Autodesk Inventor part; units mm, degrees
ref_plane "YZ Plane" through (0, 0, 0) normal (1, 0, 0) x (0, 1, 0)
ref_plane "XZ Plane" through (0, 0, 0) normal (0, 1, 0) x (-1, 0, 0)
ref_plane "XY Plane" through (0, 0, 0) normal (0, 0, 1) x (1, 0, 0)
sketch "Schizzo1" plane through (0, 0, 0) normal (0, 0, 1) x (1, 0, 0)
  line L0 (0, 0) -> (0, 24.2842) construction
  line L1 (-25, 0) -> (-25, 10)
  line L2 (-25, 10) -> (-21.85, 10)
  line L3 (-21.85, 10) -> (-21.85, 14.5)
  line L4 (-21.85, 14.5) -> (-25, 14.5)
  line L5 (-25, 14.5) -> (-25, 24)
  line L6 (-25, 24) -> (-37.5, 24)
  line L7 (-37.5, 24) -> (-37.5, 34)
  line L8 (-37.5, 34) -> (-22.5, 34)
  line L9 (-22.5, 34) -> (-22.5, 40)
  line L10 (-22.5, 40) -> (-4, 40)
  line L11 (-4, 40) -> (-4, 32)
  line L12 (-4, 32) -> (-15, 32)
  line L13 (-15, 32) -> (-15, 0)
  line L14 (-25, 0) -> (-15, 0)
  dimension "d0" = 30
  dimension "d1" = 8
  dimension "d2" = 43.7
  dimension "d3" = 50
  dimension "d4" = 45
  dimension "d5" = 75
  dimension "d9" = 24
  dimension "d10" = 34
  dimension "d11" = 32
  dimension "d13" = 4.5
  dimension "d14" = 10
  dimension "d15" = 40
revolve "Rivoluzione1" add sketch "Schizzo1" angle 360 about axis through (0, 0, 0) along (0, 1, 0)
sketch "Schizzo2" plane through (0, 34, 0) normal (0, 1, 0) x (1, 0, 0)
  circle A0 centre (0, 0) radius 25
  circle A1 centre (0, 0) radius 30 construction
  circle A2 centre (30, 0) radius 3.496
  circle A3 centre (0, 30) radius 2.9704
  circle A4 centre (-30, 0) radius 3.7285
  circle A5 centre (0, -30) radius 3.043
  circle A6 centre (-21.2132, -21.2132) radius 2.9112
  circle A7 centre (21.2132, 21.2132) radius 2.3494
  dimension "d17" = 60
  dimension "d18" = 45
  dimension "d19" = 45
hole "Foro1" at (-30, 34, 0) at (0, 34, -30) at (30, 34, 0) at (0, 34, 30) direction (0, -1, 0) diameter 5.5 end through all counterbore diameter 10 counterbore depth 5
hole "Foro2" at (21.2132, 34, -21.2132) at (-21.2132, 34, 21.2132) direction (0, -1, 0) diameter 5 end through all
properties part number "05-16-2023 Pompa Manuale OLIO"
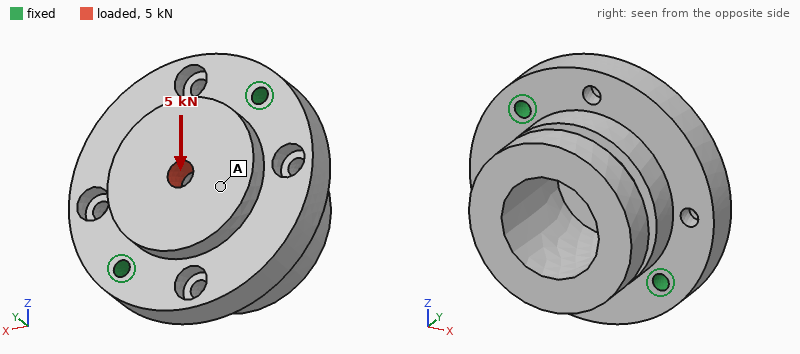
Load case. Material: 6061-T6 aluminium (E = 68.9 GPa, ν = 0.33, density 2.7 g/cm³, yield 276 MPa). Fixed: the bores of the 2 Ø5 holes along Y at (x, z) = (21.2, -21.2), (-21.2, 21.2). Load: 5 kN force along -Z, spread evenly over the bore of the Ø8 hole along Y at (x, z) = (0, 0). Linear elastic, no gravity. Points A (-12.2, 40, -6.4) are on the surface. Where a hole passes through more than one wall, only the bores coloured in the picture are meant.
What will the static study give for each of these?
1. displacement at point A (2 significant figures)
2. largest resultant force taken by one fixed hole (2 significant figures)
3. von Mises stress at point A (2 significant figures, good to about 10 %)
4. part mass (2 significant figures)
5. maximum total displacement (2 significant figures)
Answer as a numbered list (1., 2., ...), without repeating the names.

1. 14 µm
2. 2.5 kN
3. 6.7 MPa
4. 200 g
5. 26 µm
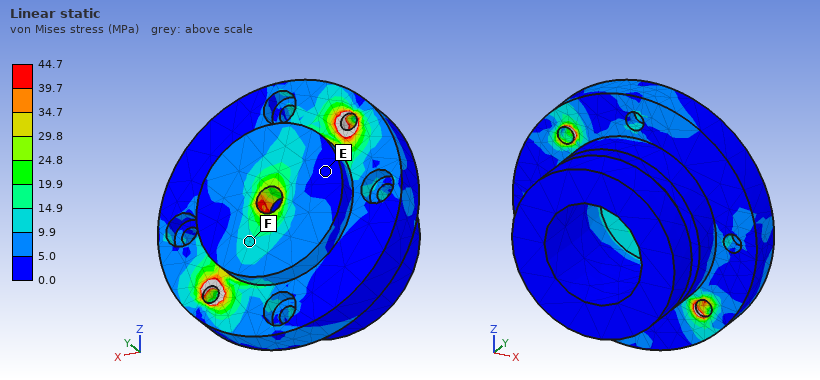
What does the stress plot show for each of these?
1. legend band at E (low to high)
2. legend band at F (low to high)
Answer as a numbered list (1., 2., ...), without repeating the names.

1. 0.0 to 5.0 MPa
2. 9.9 to 14.9 MPa
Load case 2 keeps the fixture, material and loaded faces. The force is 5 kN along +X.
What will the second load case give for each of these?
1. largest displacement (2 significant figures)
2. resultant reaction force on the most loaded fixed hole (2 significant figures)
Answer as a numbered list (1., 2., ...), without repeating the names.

1. 26 µm
2. 2.5 kN
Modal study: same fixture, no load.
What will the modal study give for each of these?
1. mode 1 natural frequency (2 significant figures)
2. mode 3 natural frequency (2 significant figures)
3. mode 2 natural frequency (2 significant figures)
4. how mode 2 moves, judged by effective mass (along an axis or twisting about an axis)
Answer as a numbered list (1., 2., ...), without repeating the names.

1. 3500 Hz
2. 12 kHz
3. 8000 Hz
4. along Y
